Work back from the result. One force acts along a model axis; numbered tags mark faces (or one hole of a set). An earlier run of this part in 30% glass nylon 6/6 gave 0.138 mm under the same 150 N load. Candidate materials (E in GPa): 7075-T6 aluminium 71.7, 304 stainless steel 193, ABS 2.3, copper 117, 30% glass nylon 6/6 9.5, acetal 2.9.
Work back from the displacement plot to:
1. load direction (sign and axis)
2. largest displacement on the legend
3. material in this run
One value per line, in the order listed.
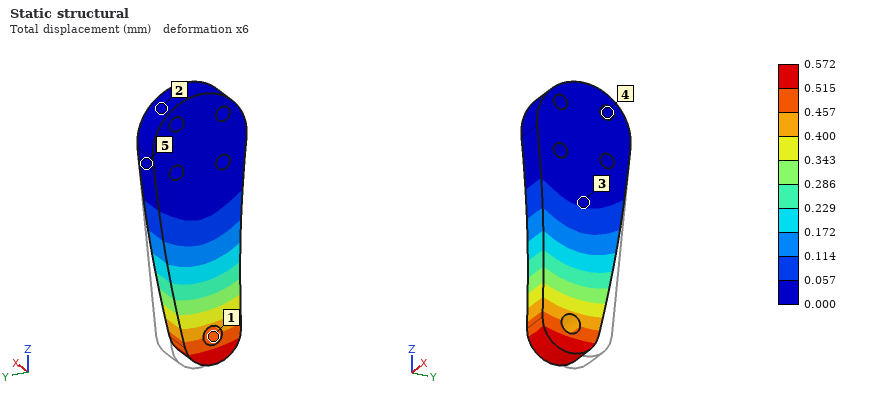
-Y
0.572 mm
ABS
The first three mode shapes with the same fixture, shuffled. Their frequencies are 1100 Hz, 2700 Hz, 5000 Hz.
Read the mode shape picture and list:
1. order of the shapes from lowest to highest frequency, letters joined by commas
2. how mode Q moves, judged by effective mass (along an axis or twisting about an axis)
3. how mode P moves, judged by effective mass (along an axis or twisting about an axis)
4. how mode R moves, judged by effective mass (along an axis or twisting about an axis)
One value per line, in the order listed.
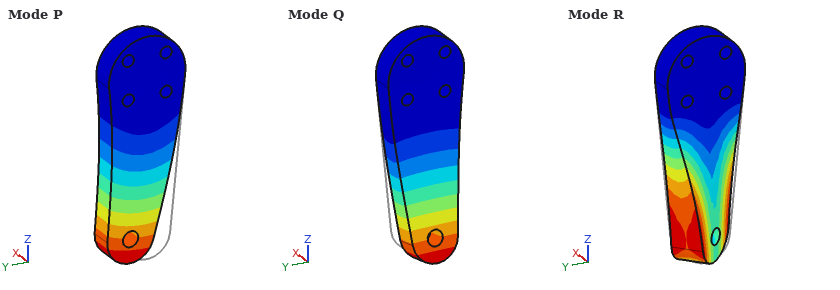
Q, P, R
along X
along Y
twisting about Z
